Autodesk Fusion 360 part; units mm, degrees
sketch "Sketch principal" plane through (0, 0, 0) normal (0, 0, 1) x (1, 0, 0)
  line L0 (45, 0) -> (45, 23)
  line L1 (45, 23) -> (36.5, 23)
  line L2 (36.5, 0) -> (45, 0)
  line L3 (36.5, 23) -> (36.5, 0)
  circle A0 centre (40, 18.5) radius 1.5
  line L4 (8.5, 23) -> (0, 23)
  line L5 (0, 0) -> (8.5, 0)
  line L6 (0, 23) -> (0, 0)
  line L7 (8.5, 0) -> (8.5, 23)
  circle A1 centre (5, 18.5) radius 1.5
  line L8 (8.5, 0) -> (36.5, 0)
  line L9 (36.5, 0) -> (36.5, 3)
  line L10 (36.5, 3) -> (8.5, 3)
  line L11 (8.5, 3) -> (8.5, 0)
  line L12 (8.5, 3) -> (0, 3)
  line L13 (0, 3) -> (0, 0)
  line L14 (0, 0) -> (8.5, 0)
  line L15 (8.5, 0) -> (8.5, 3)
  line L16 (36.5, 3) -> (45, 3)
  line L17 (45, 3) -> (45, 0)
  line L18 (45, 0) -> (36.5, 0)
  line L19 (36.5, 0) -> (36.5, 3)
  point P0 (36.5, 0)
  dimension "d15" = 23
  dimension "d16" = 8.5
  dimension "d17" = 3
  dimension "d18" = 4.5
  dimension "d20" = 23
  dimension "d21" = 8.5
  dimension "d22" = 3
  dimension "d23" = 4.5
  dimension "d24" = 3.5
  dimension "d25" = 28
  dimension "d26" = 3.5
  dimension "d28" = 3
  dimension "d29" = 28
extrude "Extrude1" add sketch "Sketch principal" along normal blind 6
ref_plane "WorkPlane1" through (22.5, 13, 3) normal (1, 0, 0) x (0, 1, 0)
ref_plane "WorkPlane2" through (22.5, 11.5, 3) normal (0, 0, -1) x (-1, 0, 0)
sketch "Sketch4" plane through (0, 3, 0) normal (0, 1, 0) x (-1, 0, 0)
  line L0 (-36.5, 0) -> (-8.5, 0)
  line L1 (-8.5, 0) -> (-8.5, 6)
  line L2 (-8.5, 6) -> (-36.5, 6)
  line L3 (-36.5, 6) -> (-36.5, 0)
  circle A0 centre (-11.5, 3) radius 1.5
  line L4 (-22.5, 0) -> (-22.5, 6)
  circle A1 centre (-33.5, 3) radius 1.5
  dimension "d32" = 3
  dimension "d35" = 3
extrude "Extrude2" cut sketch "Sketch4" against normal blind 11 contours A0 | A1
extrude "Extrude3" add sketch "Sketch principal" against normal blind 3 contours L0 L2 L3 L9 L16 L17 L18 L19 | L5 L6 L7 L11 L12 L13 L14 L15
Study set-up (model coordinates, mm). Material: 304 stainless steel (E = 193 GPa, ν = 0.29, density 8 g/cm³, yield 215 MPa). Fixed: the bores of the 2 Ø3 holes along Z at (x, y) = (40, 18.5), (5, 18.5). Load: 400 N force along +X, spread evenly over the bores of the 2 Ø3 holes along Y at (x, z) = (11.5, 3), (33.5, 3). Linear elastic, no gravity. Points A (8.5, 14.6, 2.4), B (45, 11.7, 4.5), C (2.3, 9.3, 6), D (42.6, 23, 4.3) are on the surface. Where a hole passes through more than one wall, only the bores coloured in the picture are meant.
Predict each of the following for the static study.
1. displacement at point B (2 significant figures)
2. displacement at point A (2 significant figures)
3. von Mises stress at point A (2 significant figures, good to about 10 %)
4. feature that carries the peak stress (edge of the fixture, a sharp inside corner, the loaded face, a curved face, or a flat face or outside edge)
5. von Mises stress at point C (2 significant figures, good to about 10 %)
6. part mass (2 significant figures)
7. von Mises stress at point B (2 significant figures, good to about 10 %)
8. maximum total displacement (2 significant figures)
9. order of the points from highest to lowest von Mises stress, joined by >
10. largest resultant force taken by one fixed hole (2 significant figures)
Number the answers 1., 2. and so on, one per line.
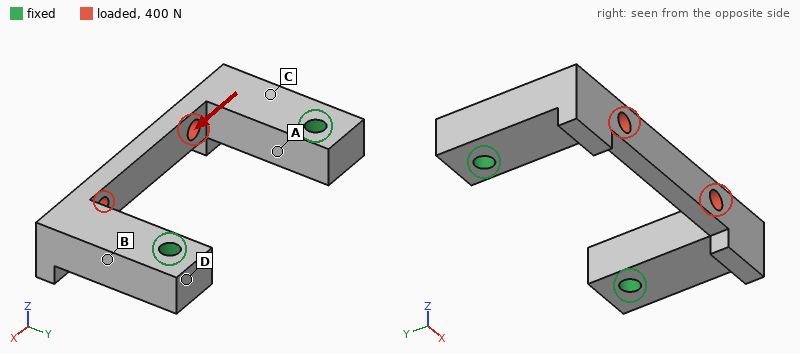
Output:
1. 3.3 µm
2. 1.7 µm
3. 34 MPa
4. edge of the fixture
5. 12 MPa
6. 23 g
7. 24 MPa
8. 9.8 µm
9. A > B > C > D
10. 200 N
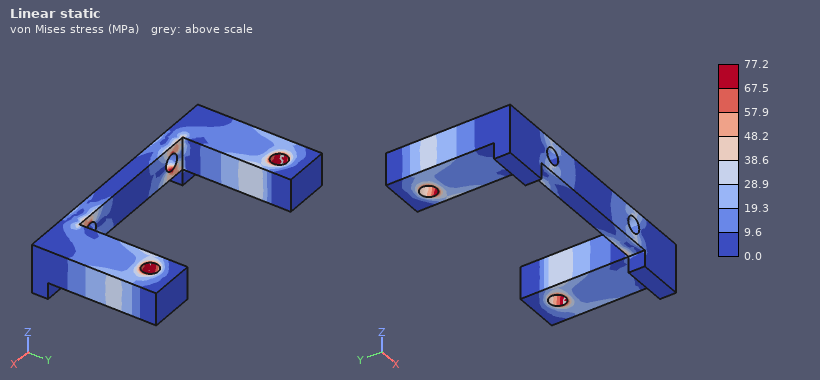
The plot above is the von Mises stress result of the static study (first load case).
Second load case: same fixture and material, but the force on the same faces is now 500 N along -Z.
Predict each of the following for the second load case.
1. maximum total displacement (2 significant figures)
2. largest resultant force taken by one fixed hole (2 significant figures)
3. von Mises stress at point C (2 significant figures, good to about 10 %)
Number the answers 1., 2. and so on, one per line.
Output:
1. 27 µm
2. 250 N
3. 44 MPa
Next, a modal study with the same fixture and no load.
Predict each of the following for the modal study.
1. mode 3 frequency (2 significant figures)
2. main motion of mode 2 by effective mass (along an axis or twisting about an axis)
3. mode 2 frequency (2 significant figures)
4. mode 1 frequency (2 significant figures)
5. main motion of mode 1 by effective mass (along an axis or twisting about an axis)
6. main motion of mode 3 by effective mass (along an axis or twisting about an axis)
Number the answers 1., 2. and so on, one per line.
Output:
1. 12 kHz
2. along X
3. 10 kHz
4. 8700 Hz
5. along Z
6. twisting about Y
